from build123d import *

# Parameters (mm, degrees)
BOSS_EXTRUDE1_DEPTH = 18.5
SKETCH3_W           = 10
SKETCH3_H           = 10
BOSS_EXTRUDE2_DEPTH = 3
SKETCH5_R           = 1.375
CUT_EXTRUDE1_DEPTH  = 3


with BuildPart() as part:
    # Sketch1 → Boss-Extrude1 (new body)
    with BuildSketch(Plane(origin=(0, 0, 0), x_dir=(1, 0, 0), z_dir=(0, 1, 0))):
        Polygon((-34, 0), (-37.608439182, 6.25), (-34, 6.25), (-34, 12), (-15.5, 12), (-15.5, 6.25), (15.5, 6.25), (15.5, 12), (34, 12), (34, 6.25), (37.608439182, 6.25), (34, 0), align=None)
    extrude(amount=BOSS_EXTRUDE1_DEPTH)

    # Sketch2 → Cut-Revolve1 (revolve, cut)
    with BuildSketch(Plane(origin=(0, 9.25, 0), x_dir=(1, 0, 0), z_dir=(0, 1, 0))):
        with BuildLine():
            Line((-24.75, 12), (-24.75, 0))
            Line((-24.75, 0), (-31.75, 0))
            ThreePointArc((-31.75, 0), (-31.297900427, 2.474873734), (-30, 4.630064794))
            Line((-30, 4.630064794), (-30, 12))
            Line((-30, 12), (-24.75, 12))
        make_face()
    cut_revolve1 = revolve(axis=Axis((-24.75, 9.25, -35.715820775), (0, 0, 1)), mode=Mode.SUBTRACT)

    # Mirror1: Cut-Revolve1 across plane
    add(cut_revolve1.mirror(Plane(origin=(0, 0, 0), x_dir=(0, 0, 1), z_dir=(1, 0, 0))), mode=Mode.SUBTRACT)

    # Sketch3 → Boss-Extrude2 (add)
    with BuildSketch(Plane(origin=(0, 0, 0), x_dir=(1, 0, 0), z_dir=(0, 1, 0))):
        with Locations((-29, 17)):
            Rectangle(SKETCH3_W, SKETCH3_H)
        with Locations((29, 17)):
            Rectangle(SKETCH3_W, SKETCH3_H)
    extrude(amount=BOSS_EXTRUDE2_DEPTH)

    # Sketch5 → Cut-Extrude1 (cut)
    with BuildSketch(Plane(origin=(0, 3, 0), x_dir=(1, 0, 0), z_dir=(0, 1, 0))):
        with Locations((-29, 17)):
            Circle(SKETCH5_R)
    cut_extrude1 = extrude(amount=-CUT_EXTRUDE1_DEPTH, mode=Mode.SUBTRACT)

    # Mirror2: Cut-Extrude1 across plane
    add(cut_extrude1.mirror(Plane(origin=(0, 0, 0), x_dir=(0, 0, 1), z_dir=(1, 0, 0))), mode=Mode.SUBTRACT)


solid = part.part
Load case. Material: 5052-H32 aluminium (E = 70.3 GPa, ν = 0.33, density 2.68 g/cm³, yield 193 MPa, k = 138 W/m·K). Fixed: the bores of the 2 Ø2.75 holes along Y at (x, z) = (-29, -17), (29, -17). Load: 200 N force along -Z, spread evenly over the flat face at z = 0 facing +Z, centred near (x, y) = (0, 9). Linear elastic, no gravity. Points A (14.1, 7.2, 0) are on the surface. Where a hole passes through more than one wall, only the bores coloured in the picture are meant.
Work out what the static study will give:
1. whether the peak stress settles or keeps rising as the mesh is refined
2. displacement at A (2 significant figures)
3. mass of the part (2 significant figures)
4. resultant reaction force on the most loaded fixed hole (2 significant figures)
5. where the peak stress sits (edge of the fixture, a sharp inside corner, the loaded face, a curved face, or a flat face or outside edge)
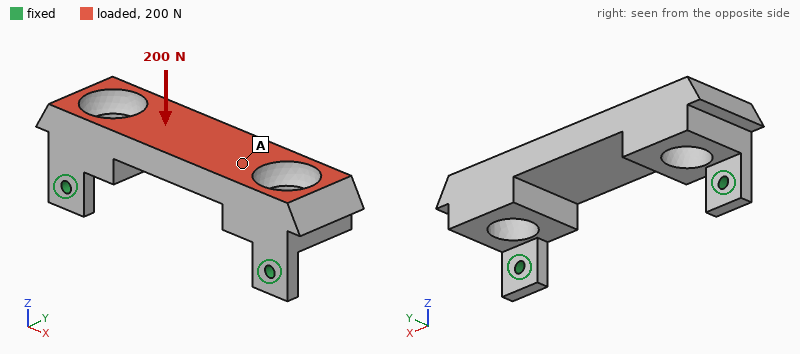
keeps rising
47 µm
28 g
120 N
edge of the fixture
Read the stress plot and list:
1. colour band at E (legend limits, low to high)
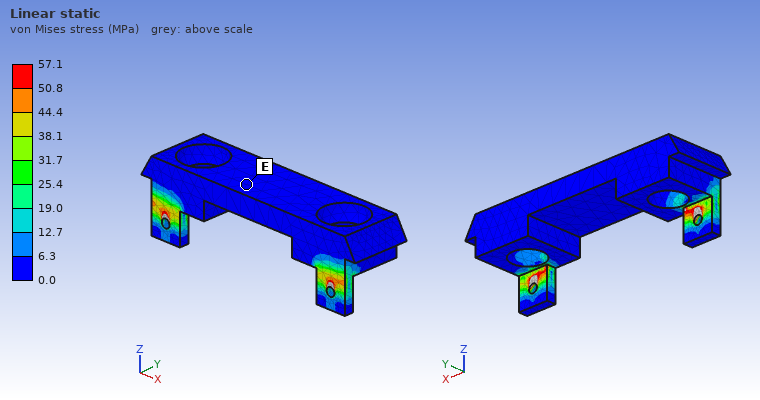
0.0 to 6.3 MPa
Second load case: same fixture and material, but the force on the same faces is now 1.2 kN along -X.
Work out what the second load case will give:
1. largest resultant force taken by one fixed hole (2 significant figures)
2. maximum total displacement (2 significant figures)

680 N
28 µm
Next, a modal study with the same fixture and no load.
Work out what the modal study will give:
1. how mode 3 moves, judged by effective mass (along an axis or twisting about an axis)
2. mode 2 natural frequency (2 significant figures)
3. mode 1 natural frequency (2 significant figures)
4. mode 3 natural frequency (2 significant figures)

along X
5300 Hz
1600 Hz
7900 Hz
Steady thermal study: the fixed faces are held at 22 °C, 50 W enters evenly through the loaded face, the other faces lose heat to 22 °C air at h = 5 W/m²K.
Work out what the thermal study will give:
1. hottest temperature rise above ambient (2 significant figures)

74 K
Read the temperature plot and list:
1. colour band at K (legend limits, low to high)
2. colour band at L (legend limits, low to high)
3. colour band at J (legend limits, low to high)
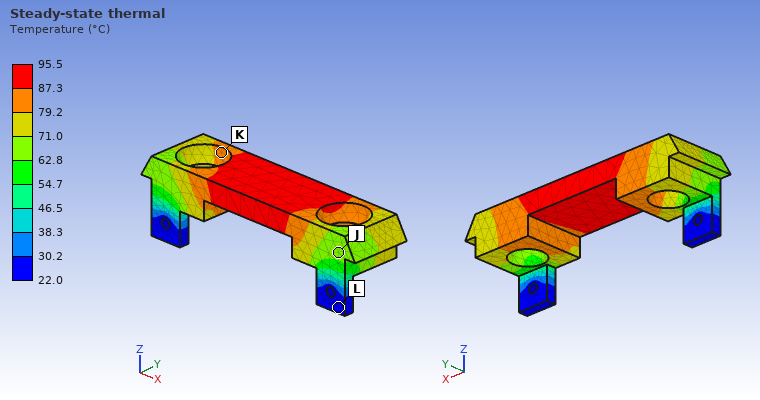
79.2 to 87.3 °C
22.0 to 30.2 °C
62.8 to 71.0 °C
